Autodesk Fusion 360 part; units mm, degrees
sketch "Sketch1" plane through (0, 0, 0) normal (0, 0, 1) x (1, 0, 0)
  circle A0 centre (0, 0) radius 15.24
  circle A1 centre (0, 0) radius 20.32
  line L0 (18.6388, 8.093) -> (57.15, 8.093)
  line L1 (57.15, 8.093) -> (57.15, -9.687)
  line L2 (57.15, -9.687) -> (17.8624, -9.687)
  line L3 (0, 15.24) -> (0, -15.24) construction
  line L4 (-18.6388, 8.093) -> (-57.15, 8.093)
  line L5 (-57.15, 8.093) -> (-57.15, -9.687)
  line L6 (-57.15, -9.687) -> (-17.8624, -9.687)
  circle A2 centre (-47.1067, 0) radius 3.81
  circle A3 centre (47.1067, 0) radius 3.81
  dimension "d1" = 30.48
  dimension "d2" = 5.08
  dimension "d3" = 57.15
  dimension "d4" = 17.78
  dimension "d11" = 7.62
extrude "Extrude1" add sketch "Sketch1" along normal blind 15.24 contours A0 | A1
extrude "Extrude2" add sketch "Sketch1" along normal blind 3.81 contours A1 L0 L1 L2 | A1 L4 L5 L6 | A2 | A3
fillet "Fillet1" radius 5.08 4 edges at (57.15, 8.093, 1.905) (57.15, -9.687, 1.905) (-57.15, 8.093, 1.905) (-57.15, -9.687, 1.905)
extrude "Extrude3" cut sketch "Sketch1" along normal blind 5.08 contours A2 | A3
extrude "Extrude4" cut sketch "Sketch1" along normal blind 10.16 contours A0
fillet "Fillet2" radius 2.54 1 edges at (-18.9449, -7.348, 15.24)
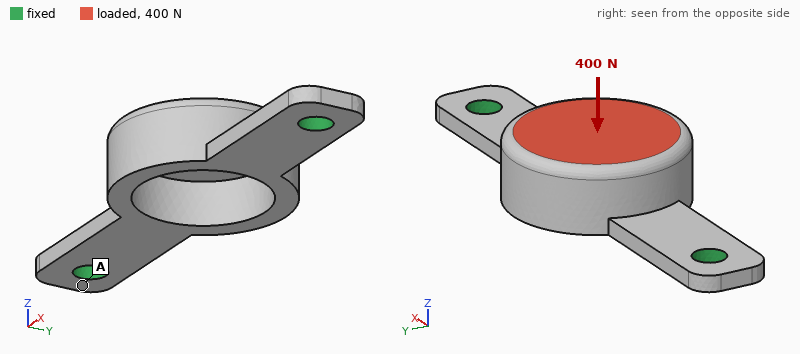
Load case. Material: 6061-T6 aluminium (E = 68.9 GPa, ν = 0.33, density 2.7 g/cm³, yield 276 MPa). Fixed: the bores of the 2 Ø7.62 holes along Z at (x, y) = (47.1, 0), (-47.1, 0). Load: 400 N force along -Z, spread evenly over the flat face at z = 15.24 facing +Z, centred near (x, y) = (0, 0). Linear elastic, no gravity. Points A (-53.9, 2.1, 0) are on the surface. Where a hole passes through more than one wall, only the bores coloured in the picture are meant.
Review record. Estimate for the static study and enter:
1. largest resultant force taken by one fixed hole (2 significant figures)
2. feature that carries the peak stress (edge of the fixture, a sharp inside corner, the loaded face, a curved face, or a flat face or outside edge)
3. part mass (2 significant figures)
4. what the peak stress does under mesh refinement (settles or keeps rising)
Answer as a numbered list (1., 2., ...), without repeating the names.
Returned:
1. 360 N
2. edge of the fixture
3. 45 g
4. keeps rising
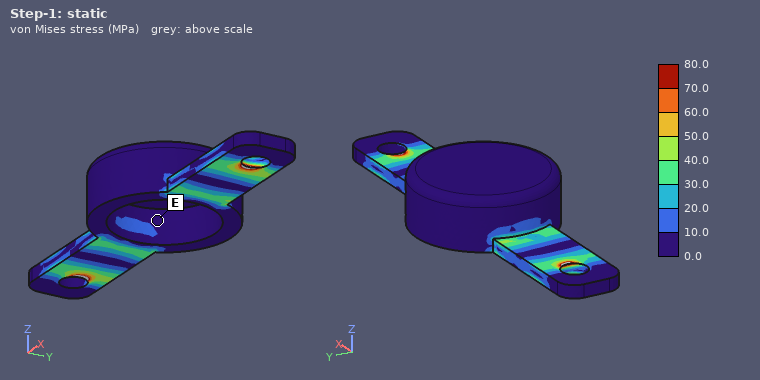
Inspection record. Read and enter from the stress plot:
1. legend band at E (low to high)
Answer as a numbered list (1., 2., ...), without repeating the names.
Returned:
1. 0.0 to 10.0 MPa
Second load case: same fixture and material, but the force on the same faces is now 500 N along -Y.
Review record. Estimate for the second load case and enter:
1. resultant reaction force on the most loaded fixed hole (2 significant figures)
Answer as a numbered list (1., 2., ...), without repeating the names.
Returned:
1. 250 N
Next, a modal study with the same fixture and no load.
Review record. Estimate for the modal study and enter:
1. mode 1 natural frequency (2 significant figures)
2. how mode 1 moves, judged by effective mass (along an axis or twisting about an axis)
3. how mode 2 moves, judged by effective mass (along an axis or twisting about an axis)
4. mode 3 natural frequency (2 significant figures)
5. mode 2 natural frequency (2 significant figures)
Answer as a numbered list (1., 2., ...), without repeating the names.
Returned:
1. 1600 Hz
2. along Y
3. along Z
4. 4600 Hz
5. 2100 Hz
